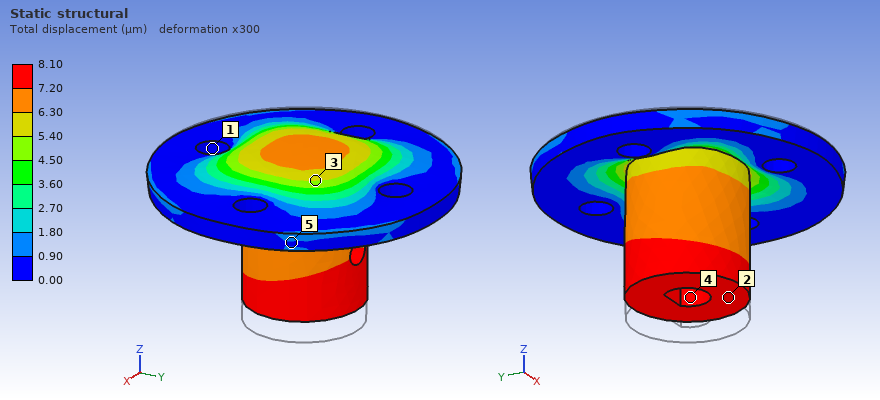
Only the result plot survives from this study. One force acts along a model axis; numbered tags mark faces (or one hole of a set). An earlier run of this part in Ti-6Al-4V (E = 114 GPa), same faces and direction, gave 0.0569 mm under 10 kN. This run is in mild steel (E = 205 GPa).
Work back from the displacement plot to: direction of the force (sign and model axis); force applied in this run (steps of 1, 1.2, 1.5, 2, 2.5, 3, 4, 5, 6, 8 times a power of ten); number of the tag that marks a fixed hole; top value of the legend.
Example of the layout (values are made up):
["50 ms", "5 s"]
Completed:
["+Z", "2.5 kN", "1", "8.10 µm"]
